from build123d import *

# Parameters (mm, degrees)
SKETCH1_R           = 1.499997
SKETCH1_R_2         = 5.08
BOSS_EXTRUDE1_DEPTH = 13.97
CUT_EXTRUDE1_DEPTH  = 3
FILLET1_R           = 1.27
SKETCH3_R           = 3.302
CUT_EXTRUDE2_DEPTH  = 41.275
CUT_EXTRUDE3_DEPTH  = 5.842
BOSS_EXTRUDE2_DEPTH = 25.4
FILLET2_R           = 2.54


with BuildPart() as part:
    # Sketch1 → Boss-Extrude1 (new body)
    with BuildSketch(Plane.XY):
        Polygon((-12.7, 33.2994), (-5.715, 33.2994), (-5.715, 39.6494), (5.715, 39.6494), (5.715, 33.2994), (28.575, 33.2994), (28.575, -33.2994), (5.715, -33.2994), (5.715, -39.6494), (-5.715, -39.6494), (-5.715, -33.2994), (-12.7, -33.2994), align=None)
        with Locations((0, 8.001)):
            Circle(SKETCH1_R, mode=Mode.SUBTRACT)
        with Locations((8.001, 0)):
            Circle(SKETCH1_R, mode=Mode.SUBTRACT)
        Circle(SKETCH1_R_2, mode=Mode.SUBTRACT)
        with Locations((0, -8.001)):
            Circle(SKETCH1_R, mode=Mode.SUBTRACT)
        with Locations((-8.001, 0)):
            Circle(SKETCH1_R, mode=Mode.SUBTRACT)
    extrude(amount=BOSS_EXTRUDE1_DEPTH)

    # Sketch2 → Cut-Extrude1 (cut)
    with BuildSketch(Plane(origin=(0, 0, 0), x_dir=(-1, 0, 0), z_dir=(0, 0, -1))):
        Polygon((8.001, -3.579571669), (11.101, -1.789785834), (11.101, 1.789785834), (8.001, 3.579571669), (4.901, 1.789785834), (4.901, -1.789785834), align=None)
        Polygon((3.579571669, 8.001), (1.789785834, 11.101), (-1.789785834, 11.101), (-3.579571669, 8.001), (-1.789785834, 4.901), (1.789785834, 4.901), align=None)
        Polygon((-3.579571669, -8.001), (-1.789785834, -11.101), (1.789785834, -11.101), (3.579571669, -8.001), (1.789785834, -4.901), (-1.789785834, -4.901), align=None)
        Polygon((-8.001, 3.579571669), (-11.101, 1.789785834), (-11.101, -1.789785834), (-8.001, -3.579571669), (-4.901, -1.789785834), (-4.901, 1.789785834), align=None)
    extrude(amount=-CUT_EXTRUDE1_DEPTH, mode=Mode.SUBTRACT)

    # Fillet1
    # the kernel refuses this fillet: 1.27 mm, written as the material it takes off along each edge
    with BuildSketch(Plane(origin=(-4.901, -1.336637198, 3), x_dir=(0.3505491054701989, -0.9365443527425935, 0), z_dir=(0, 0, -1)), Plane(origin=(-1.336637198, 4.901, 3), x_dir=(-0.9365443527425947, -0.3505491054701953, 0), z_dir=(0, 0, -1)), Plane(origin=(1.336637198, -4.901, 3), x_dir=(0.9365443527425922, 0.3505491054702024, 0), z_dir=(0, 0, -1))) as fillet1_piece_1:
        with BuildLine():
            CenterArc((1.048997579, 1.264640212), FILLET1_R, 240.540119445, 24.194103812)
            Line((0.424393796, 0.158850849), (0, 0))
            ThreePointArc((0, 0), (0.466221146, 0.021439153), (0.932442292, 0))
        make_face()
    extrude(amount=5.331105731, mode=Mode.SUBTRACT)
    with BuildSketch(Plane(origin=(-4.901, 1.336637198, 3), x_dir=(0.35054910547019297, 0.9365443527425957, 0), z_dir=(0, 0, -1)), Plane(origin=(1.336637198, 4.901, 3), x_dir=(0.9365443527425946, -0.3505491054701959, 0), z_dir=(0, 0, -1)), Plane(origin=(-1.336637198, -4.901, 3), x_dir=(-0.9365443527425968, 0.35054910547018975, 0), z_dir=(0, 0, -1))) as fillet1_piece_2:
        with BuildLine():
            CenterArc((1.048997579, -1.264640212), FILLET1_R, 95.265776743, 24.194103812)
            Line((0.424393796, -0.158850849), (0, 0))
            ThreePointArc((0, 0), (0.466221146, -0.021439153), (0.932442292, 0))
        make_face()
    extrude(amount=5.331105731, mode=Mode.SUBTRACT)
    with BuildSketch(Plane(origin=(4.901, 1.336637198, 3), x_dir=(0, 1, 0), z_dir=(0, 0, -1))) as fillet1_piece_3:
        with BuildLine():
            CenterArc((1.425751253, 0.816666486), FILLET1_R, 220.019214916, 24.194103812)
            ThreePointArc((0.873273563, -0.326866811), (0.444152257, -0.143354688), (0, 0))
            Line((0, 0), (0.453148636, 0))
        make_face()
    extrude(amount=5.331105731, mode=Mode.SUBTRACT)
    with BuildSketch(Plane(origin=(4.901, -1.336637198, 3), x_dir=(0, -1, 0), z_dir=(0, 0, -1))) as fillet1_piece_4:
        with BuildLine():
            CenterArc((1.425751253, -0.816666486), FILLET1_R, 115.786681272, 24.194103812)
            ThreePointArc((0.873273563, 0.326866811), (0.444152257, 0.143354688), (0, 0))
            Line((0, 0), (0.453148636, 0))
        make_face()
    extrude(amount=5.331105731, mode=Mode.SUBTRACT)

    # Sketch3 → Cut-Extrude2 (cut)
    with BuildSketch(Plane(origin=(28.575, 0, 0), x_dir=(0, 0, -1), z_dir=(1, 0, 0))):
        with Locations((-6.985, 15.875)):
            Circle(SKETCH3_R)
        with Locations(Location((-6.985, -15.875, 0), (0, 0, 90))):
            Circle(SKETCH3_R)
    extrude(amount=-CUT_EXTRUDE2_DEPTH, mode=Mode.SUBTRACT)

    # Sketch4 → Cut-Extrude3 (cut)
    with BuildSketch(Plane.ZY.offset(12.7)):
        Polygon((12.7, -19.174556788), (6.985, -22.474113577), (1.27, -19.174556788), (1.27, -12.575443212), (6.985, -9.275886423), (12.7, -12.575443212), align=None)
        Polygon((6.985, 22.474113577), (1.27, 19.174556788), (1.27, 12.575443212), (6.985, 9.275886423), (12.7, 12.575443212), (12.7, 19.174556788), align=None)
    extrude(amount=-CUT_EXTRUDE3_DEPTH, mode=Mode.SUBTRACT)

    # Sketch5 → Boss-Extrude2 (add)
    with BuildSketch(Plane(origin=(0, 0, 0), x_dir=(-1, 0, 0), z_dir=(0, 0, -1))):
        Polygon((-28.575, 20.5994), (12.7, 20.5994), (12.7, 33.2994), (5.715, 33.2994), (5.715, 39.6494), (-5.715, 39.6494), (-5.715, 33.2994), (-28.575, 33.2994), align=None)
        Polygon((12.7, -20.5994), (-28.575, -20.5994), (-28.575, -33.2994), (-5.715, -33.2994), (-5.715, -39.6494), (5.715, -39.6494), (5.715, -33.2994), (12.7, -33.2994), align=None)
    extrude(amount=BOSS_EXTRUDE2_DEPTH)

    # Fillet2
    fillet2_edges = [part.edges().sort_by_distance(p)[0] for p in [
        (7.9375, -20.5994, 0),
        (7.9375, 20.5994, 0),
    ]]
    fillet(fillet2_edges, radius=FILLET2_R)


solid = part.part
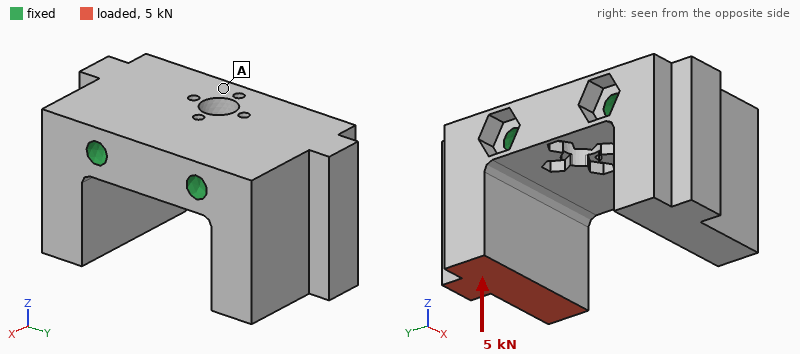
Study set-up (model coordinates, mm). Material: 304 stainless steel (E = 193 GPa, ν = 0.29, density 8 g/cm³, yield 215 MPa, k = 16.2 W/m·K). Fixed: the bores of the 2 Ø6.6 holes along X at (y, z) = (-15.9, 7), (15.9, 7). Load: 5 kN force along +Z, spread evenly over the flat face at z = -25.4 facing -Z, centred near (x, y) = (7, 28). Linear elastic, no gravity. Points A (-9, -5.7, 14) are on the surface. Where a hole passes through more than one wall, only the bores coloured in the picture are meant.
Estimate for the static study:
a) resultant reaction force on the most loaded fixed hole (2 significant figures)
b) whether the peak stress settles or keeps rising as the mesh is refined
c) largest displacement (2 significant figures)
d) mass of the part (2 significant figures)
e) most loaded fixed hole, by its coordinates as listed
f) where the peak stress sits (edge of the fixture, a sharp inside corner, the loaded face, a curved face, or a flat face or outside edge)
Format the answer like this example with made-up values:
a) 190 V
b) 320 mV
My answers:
a) 5.4 kN
b) keeps rising
c) 14 µm
d) 520 g
e) (15.9, 7)
f) edge of the fixture
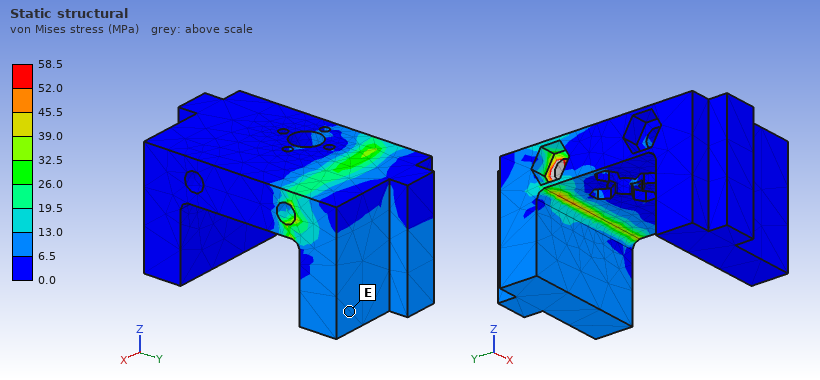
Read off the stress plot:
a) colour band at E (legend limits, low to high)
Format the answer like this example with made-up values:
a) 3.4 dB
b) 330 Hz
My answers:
a) 6.5 to 13.0 MPa
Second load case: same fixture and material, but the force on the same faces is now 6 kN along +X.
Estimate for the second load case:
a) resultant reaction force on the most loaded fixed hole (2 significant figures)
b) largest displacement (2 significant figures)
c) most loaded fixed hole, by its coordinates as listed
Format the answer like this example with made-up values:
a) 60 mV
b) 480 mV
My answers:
a) 6.0 kN
b) 25 µm
c) (15.9, 7)
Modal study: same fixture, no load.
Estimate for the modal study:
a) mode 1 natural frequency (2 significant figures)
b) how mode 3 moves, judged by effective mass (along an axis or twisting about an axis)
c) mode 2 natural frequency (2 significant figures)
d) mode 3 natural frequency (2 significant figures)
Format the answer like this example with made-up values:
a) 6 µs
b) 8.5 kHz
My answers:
a) 6500 Hz
b) along X
c) 6600 Hz
d) 11 kHz
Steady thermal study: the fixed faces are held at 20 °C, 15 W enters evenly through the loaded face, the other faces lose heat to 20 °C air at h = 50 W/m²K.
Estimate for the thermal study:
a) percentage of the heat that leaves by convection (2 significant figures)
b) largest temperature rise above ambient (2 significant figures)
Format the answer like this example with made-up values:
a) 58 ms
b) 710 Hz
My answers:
a) 34 %
b) 46 K
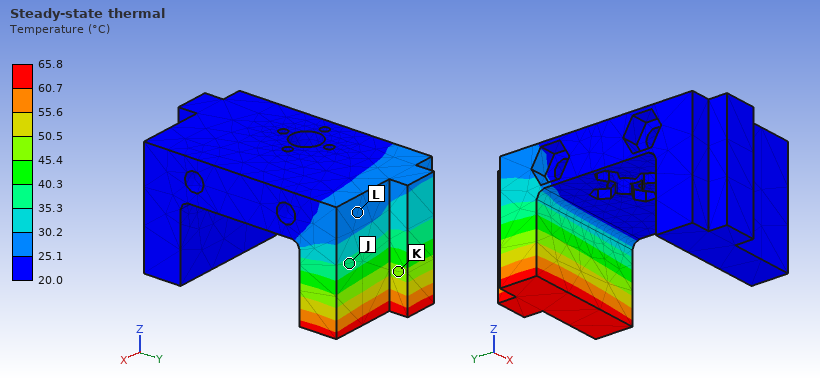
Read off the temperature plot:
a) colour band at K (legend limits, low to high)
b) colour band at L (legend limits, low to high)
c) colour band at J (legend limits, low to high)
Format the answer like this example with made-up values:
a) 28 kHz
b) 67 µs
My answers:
a) 45.4 to 50.5 °C
b) 25.1 to 30.2 °C
c) 35.3 to 40.3 °C
